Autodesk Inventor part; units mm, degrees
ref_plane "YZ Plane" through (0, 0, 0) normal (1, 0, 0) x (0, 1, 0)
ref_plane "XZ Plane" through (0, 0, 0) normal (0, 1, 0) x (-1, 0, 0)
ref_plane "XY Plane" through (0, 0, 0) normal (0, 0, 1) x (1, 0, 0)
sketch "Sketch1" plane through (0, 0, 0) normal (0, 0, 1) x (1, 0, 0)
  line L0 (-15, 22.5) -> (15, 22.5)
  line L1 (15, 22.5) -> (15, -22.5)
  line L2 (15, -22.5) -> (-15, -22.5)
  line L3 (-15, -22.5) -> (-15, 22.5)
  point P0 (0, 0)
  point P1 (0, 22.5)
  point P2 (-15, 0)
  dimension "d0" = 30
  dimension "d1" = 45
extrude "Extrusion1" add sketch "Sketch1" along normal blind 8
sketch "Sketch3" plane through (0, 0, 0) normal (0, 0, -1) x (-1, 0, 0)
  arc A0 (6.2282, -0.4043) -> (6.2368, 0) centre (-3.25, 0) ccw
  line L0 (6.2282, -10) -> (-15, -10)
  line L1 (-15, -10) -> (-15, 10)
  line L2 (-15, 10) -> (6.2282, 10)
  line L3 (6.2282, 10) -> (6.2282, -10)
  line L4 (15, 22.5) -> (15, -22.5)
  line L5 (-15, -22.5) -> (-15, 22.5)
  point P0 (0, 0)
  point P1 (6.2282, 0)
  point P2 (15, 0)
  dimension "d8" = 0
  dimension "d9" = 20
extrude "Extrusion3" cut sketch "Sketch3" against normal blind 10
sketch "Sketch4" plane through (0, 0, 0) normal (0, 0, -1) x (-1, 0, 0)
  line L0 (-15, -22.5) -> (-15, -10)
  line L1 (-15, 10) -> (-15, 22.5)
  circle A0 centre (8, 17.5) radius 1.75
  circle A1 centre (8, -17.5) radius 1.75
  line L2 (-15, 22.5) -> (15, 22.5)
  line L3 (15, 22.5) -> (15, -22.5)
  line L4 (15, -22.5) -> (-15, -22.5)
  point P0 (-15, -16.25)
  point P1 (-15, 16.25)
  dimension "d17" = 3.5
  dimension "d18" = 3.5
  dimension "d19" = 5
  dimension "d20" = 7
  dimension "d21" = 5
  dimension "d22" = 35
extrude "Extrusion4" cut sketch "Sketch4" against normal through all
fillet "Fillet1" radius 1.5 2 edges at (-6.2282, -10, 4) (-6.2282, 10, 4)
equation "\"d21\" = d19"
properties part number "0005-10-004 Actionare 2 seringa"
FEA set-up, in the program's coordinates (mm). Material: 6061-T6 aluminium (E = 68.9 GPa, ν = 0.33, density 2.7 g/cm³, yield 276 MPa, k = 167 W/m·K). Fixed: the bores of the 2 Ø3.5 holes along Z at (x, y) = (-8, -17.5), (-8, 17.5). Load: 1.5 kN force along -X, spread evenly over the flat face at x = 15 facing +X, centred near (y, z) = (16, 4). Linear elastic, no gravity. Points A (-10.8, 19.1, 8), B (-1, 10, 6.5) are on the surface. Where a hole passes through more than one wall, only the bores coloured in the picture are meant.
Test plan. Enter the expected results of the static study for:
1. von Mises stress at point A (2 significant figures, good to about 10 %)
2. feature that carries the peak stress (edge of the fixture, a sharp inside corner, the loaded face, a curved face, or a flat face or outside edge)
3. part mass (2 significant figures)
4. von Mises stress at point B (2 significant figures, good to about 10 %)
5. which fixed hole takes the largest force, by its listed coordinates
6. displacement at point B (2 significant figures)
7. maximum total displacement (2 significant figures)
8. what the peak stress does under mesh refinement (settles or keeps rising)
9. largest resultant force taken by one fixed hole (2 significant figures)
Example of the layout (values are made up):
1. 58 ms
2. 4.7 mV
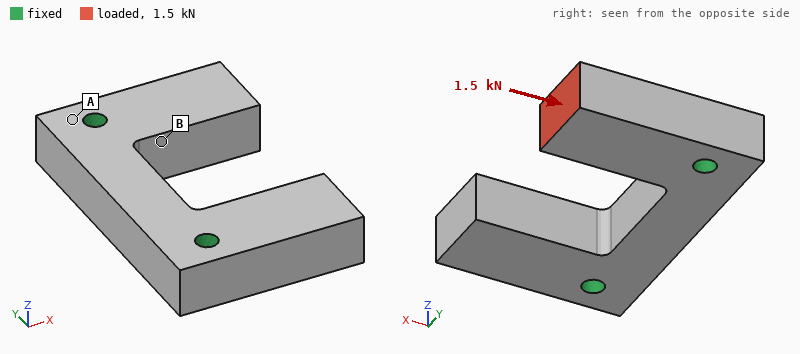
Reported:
1. 4.6 MPa
2. edge of the fixture
3. 20 g
4. 13 MPa
5. (-8, 17.5)
6. 3.1 µm
7. 7.2 µm
8. keeps rising
9. 1.5 kN
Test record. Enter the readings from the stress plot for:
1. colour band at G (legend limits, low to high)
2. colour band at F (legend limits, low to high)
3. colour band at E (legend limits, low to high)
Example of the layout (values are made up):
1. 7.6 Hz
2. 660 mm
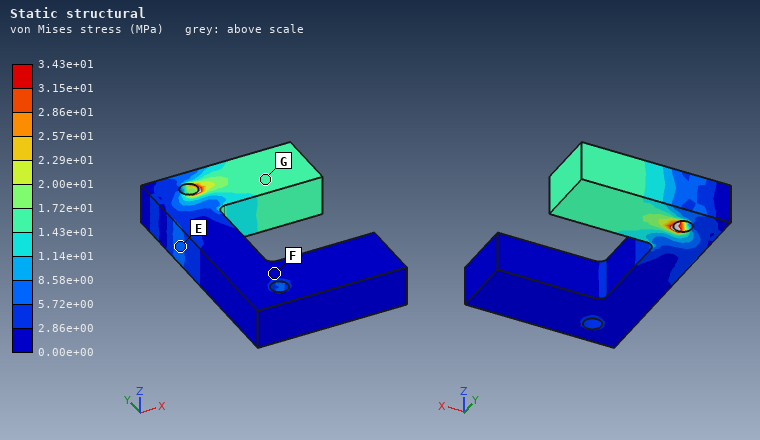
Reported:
1. 1.43e+01 to 1.72e+01 MPa
2. 0.00e+00 to 2.86e+00 MPa
3. 5.72e+00 to 8.58e+00 MPa
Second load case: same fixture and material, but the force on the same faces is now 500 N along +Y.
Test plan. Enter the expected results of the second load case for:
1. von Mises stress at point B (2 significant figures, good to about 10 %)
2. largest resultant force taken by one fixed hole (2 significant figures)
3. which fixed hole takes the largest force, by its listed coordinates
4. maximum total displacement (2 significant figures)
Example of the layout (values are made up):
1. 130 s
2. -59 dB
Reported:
1. 38 MPa
2. 710 N
3. (-8, 17.5)
4. 45 µm
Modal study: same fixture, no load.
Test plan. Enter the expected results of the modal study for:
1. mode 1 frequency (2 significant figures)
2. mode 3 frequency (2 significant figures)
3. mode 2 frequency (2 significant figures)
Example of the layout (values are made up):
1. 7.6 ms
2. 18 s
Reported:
1. 11 kHz
2. 12 kHz
3. 11 kHz
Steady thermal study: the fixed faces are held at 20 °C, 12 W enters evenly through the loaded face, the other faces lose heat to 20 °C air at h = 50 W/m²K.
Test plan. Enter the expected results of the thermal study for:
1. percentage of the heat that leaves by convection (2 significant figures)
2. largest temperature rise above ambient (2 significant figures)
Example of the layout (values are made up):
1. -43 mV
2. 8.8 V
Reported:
1. 3.4 %
2. 16 K
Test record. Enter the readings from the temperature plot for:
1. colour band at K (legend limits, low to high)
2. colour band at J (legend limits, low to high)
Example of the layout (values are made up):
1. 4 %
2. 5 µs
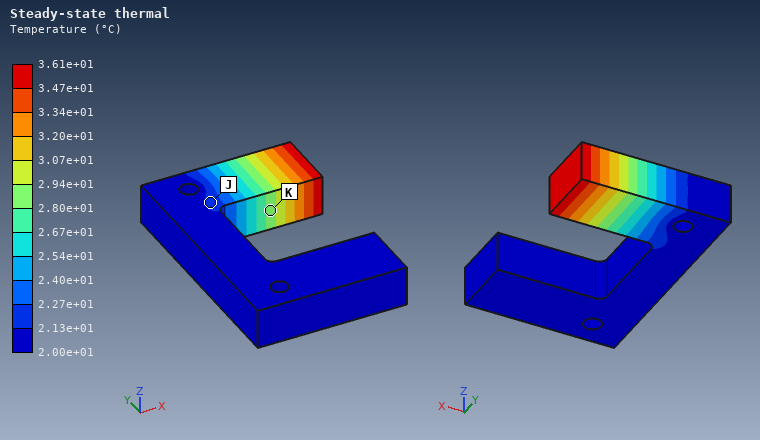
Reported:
1. 2.80e+01 to 2.94e+01 °C
2. 2.13e+01 to 2.27e+01 °C
